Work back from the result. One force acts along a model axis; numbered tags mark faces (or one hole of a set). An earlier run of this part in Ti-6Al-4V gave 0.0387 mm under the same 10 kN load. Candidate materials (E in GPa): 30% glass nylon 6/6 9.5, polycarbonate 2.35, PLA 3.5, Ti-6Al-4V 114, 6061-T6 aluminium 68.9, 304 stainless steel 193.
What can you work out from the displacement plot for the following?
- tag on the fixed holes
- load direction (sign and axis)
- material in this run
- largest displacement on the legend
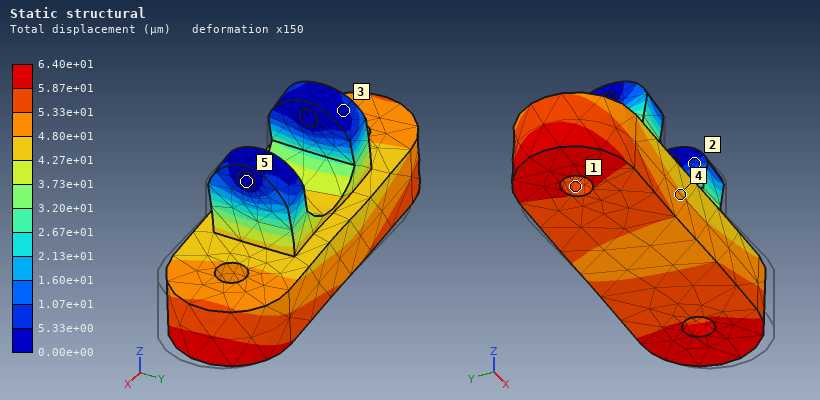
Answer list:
5
-X
6061-T6 aluminium
6.40e+01 µm
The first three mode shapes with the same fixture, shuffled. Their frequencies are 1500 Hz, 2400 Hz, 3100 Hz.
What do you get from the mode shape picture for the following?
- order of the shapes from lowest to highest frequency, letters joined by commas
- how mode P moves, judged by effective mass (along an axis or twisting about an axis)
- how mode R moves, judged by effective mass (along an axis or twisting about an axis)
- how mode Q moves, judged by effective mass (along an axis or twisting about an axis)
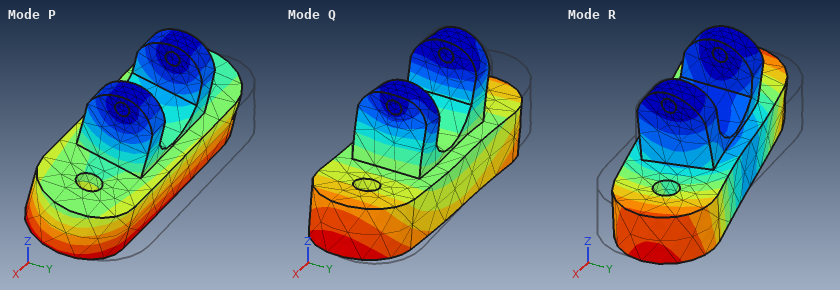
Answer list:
P, R, Q
along Y
twisting about Z
along X
